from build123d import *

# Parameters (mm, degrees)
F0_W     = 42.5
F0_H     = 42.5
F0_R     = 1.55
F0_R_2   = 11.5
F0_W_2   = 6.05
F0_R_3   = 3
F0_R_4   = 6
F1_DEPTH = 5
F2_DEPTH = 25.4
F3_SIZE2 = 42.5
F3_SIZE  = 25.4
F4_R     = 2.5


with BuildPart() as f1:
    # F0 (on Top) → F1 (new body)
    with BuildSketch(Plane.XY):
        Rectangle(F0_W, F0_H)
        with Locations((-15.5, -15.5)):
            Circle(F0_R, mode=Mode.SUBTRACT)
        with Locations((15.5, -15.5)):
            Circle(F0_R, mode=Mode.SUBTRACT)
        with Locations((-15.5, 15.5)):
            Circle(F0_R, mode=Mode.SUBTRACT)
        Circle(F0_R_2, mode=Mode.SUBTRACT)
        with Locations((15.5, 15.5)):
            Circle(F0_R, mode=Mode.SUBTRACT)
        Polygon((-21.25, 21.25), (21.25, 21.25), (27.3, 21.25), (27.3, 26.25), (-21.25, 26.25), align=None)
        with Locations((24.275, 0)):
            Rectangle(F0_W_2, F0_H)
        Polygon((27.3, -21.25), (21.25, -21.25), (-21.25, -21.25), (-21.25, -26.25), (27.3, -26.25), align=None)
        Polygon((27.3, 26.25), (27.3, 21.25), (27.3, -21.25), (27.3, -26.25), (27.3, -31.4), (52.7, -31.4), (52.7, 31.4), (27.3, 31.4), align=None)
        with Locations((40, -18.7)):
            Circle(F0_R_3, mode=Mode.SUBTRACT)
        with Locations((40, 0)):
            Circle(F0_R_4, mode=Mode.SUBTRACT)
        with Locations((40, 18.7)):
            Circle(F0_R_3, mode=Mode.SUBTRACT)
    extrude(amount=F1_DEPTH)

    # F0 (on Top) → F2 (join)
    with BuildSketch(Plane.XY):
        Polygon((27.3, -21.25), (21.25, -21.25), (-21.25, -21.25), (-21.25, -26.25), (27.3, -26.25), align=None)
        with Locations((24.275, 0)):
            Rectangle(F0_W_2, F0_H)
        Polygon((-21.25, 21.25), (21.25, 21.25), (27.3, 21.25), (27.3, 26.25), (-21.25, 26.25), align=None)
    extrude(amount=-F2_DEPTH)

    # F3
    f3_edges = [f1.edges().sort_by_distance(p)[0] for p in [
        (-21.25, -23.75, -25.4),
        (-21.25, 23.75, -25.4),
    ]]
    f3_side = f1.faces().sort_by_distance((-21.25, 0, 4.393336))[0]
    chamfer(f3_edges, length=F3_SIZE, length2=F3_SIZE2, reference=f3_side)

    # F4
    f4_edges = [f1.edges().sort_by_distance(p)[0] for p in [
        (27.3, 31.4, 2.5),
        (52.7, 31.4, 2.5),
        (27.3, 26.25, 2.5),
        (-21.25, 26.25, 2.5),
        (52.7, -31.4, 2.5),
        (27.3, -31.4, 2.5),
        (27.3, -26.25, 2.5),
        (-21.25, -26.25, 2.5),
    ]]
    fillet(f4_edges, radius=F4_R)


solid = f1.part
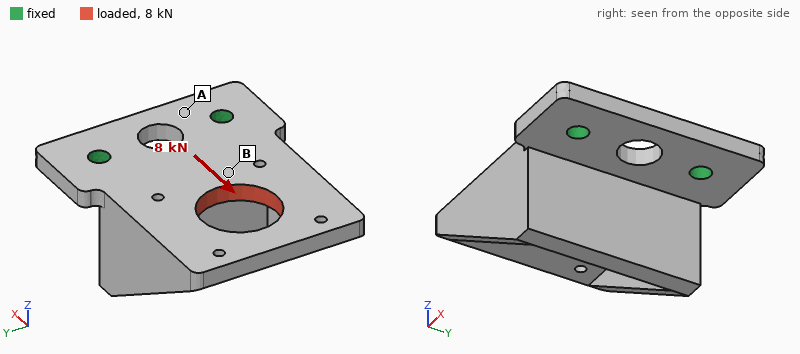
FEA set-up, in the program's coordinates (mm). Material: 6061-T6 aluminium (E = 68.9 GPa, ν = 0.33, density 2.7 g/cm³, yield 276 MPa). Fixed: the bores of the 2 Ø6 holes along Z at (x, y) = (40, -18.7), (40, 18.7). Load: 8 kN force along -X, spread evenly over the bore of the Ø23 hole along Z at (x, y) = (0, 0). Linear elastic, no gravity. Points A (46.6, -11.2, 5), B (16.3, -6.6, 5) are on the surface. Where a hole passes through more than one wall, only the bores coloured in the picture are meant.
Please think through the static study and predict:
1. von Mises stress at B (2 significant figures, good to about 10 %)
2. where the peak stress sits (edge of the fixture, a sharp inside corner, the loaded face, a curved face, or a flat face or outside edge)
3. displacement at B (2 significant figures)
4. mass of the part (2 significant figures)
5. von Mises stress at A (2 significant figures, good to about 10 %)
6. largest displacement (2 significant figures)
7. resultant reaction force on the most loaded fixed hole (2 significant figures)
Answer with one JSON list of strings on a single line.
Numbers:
["31 MPa", "a curved face", "14 µm", "84 g", "15 MPa", "53 µm", "4.0 kN"]
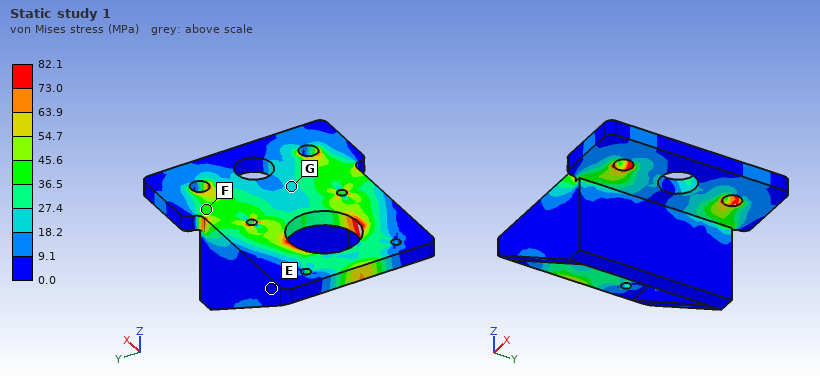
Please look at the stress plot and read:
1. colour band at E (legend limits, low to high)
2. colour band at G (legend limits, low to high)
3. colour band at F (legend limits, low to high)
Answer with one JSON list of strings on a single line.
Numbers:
["0.0 to 9.1 MPa", "18.2 to 27.4 MPa", "36.5 to 45.6 MPa"]
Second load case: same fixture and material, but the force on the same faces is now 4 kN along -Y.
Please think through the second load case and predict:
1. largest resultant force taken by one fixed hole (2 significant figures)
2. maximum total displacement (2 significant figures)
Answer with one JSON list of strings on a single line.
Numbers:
["4.3 kN", "91 µm"]
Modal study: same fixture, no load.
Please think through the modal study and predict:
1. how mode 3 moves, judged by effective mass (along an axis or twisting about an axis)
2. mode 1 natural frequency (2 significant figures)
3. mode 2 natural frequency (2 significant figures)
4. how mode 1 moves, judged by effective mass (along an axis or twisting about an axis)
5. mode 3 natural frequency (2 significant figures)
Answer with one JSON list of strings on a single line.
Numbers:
["along Y", "1100 Hz", "3100 Hz", "along Z", "6300 Hz"]
